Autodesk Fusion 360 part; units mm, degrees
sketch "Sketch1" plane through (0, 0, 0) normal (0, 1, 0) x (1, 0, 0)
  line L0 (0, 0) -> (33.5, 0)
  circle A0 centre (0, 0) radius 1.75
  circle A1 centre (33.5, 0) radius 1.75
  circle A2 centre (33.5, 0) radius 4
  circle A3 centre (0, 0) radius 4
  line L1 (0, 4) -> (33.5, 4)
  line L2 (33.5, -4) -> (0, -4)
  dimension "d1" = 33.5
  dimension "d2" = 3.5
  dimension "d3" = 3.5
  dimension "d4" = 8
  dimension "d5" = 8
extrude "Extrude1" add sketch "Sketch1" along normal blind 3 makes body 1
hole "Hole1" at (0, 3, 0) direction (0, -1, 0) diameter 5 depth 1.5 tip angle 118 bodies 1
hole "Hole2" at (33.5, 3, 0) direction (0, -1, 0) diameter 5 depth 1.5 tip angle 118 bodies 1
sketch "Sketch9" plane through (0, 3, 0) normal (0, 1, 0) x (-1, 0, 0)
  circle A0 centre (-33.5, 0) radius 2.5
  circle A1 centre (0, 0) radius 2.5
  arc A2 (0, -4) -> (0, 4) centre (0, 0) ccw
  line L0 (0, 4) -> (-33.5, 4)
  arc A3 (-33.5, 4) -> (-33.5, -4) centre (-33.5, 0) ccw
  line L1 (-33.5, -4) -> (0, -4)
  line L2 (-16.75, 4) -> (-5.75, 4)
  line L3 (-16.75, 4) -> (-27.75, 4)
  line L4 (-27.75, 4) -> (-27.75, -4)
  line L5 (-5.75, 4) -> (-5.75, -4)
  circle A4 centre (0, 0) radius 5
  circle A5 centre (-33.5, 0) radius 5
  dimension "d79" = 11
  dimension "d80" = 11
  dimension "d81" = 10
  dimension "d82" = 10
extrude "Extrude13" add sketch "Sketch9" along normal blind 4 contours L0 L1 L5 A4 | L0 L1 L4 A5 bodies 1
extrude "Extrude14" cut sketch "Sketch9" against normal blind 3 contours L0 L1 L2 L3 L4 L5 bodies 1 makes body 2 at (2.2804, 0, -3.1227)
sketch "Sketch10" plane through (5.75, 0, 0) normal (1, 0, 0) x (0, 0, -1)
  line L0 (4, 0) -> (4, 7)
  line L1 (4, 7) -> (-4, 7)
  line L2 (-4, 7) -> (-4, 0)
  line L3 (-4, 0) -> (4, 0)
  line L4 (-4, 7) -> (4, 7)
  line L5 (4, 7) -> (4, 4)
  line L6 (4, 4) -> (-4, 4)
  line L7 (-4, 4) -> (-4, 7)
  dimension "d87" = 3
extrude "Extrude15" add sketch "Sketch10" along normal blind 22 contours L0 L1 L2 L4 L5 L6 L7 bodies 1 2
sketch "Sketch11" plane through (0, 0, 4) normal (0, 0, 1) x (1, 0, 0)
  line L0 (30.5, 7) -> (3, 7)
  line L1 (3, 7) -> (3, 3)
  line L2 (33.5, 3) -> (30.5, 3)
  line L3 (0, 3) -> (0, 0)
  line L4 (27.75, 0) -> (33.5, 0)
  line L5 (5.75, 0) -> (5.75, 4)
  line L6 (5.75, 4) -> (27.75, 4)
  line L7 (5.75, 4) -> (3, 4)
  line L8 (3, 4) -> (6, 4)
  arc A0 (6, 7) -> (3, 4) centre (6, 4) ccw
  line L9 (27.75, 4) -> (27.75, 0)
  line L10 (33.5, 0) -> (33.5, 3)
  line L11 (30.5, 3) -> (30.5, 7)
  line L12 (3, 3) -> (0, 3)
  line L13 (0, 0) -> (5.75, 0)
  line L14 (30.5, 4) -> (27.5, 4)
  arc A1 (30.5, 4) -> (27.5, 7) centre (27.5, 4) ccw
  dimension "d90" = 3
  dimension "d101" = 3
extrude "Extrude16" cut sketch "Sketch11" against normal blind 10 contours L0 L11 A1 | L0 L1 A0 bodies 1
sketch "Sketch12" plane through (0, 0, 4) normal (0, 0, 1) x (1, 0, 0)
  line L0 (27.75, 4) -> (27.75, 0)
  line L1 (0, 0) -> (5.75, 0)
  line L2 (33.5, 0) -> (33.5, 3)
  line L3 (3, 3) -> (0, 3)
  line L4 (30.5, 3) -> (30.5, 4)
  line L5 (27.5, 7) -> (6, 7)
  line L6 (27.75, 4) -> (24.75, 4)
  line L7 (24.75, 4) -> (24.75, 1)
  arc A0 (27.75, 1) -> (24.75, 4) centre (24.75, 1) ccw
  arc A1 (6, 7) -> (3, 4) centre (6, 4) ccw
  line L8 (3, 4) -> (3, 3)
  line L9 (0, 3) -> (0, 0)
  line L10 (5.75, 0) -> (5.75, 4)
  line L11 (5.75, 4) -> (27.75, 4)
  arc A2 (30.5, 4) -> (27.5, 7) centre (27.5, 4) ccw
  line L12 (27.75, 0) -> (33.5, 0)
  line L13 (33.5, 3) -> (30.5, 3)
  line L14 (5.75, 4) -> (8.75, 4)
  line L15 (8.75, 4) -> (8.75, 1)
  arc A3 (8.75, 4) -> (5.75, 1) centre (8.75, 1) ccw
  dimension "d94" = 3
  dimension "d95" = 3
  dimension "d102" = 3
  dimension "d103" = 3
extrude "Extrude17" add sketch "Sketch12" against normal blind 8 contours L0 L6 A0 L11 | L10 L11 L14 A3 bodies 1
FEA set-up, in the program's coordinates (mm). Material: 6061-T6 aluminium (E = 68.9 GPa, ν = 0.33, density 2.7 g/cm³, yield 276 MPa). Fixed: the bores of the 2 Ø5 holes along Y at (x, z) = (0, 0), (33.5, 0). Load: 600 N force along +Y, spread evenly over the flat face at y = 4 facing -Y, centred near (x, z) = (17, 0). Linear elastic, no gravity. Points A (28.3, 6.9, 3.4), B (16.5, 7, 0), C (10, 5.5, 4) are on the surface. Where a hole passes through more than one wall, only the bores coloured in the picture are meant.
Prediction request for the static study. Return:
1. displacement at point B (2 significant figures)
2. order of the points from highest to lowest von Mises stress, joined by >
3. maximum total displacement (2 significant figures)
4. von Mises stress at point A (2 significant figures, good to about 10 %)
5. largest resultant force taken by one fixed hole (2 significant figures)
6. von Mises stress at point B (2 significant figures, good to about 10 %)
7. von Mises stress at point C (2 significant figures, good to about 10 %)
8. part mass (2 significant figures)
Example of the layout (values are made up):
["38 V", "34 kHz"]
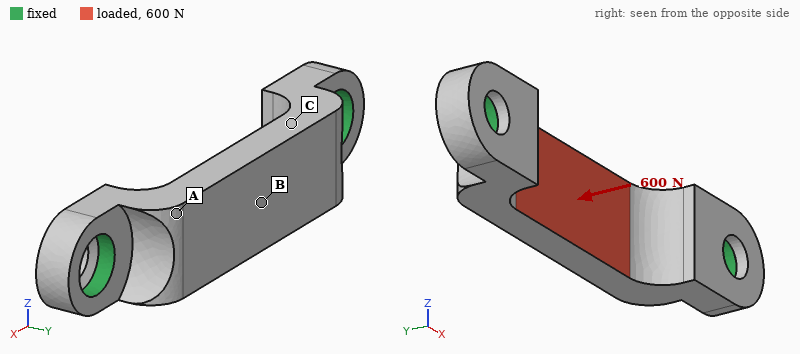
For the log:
["32 µm", "B > C > A", "34 µm", "15 MPa", "570 N", "89 MPa", "45 MPa", "2.6 g"]
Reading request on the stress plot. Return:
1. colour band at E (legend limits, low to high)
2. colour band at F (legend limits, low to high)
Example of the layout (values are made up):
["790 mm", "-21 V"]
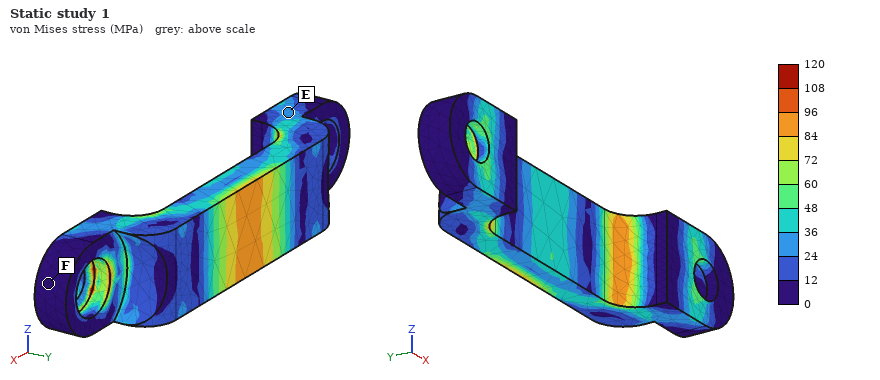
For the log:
["24 to 36 MPa", "0 to 12 MPa"]
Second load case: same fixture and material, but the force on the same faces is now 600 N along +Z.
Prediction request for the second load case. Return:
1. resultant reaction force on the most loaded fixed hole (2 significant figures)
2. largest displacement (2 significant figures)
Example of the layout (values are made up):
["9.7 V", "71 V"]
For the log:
["300 N", "24 µm"]
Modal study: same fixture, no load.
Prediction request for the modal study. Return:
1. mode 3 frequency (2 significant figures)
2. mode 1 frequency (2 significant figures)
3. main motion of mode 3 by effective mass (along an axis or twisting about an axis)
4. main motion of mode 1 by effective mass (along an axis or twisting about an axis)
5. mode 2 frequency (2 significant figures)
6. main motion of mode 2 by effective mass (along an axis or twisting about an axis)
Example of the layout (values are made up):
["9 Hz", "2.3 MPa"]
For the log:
["29 kHz", "20 kHz", "along X", "along Z", "22 kHz", "along Y"]
